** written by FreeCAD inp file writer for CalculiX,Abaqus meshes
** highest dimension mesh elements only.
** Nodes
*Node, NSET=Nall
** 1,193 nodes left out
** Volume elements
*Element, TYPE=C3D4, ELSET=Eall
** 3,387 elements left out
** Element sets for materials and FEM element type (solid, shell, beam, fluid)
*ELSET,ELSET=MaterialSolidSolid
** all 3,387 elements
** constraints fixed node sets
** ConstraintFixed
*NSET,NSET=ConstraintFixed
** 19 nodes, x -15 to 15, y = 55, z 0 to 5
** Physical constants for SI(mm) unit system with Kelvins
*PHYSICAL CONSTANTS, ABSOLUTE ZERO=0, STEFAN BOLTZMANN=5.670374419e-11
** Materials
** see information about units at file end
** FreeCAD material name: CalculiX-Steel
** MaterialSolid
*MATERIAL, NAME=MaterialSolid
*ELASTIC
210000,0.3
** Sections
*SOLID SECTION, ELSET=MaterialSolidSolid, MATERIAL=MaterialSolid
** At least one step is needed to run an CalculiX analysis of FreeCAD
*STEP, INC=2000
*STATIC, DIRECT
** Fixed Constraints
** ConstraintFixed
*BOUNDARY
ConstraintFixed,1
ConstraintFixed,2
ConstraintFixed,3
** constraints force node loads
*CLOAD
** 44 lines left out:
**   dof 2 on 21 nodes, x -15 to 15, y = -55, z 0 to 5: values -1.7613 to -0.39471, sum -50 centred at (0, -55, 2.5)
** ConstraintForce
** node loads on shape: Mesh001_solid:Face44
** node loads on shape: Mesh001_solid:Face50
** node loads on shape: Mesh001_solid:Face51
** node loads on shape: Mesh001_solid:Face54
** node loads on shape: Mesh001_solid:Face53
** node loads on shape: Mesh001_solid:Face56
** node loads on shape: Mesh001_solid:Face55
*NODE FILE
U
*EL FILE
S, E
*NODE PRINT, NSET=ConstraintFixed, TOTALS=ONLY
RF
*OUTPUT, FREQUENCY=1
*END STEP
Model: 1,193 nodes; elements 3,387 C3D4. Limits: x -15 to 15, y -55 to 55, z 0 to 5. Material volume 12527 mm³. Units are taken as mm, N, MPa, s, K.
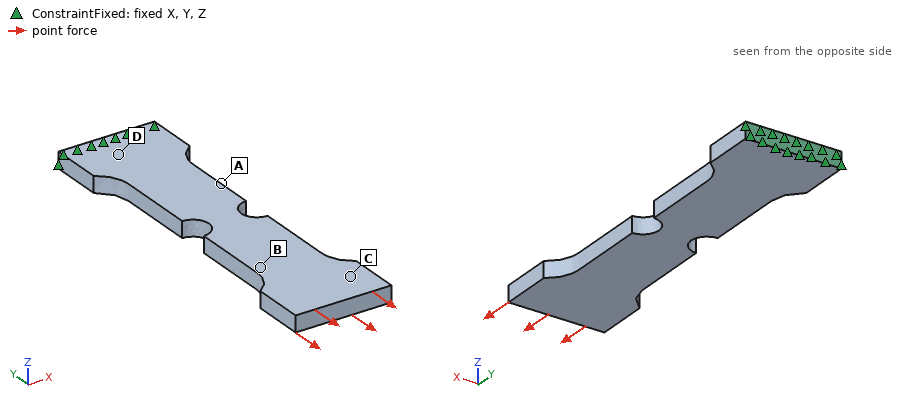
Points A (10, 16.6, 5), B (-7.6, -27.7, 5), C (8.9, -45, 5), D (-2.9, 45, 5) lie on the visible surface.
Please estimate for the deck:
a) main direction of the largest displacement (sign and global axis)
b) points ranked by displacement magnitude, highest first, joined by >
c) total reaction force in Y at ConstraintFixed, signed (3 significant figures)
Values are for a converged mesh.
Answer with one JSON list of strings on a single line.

["-Y", "C > B > A > D", "50.0 N"]
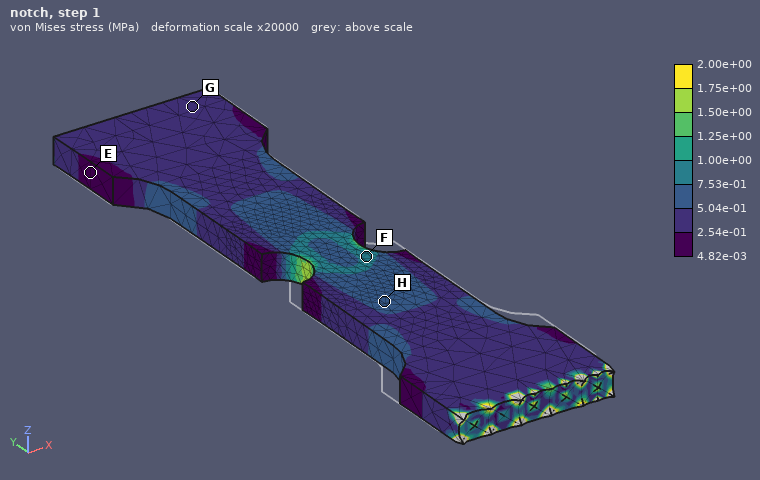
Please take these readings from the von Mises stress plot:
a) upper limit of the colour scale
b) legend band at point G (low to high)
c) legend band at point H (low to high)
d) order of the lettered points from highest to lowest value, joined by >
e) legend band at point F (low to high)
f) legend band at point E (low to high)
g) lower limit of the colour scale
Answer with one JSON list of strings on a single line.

["2.00e+00 MPa", "2.54e-01 to 5.04e-01 MPa", "5.04e-01 to 7.53e-01 MPa", "F > H > G > E", "7.53e-01 to 1.00e+00 MPa", "4.82e-03 to 2.54e-01 MPa", "4.82e-03 MPa"]
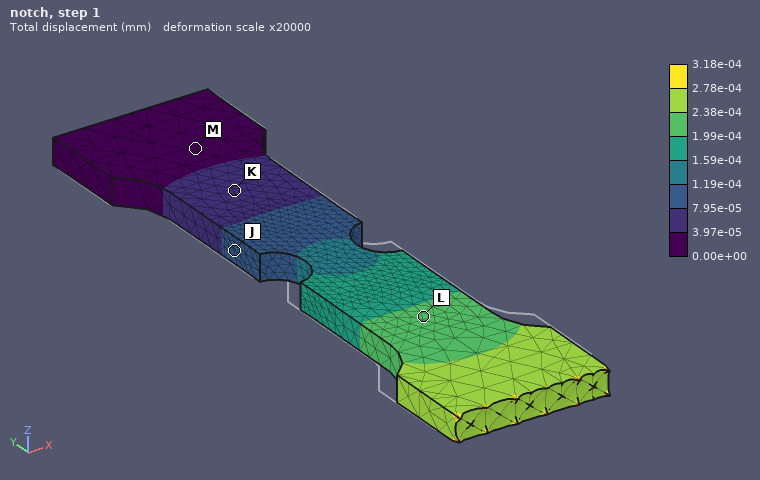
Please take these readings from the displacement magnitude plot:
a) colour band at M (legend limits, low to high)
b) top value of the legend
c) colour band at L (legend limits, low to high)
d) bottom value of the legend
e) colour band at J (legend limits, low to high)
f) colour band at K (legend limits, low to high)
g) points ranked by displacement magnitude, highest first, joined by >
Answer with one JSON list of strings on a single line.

["0.00e+00 to 3.97e-05 mm", "3.18e-04 mm", "1.99e-04 to 2.38e-04 mm", "0.00e+00 mm", "7.95e-05 to 1.19e-04 mm", "3.97e-05 to 7.95e-05 mm", "L > J > K > M"]
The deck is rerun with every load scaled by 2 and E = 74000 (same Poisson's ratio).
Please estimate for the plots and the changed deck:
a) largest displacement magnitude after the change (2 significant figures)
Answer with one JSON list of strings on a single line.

["0.0018 mm"]
